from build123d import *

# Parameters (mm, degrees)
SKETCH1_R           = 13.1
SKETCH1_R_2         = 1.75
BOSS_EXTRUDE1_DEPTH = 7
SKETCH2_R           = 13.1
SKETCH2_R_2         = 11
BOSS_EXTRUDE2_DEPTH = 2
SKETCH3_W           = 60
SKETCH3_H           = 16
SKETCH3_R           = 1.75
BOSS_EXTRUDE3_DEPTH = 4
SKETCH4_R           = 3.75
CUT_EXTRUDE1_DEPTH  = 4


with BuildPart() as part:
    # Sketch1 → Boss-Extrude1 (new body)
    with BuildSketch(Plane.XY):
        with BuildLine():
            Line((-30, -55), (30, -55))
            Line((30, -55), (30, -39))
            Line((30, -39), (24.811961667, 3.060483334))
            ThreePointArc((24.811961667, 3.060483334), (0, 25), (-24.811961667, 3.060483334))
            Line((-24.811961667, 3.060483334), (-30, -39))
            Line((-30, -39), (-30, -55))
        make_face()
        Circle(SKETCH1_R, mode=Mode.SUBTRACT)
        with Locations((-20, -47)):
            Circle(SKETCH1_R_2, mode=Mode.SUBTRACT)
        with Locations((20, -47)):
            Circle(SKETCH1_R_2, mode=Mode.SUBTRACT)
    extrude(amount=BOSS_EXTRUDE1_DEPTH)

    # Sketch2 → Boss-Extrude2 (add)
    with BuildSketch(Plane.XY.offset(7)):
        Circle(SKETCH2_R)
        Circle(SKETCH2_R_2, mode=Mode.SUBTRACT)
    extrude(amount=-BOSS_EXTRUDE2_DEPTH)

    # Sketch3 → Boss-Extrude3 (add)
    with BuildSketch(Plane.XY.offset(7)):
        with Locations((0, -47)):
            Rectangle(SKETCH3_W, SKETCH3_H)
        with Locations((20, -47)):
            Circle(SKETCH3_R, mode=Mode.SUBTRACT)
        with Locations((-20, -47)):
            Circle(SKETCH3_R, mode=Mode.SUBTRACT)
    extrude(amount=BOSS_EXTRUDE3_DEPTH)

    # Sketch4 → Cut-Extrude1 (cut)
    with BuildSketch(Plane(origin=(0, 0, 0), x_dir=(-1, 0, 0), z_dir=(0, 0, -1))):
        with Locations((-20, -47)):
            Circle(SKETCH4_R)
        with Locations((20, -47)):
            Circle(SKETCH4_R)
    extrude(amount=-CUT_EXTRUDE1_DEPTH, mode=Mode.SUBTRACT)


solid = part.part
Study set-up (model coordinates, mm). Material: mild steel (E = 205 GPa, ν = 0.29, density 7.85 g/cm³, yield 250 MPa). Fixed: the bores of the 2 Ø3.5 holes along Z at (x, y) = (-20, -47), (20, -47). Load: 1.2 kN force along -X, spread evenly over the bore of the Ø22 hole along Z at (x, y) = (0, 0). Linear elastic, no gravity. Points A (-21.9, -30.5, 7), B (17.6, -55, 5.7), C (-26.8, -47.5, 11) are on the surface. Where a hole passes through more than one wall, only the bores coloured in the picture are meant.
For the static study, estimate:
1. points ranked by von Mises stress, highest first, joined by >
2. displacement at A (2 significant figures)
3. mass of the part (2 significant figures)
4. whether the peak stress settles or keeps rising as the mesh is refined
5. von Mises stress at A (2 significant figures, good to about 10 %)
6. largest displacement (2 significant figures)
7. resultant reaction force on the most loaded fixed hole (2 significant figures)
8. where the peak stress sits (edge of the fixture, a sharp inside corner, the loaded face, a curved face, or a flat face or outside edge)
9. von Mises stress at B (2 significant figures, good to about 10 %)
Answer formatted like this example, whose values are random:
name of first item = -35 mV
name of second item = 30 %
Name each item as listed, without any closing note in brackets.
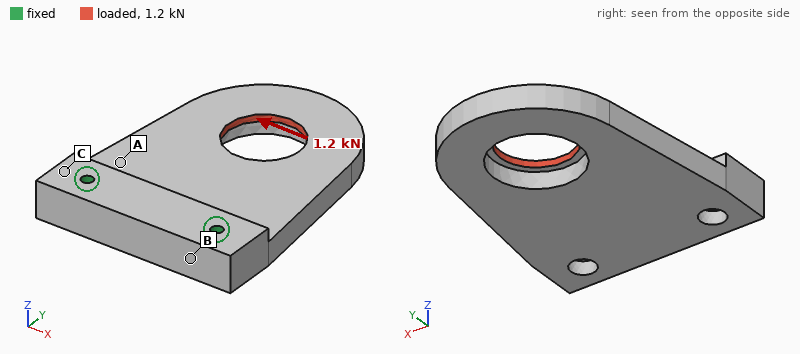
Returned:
points ranked by von Mises stress, highest first, joined by > = A > B > C
displacement at A = 2.9 µm
mass of the part = 220 g
whether the peak stress settles or keeps rising as the mesh is refined = keeps rising
von Mises stress at A = 11 MPa
largest displacement = 12 µm
resultant reaction force on the most loaded fixed hole = 1.5 kN
where the peak stress sits = edge of the fixture
von Mises stress at B = 7.7 MPa
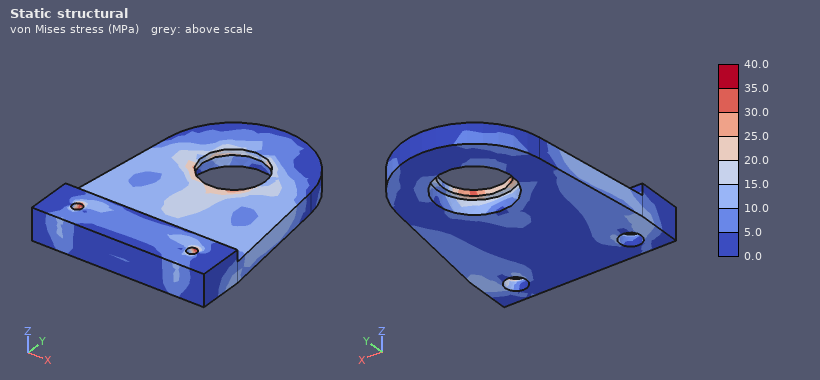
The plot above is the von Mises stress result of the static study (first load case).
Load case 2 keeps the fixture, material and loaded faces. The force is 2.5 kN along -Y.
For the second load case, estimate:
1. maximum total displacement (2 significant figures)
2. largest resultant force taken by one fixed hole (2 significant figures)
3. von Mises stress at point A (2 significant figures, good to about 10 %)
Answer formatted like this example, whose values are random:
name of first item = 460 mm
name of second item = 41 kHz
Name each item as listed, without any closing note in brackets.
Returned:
maximum total displacement = 36 µm
largest resultant force taken by one fixed hole = 1.3 kN
von Mises stress at point A = 20 MPa
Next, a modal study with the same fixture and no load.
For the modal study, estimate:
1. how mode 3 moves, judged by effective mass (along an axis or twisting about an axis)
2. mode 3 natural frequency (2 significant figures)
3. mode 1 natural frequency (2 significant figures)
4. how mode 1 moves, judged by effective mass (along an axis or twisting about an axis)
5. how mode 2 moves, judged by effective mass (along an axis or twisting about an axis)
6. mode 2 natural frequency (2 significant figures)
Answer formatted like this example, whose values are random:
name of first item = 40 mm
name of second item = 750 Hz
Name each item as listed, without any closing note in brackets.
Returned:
how mode 3 moves, judged by effective mass = along Z
mode 3 natural frequency = 6100 Hz
mode 1 natural frequency = 1400 Hz
how mode 1 moves, judged by effective mass = along Z
how mode 2 moves, judged by effective mass = twisting about Y
mode 2 natural frequency = 4200 Hz
